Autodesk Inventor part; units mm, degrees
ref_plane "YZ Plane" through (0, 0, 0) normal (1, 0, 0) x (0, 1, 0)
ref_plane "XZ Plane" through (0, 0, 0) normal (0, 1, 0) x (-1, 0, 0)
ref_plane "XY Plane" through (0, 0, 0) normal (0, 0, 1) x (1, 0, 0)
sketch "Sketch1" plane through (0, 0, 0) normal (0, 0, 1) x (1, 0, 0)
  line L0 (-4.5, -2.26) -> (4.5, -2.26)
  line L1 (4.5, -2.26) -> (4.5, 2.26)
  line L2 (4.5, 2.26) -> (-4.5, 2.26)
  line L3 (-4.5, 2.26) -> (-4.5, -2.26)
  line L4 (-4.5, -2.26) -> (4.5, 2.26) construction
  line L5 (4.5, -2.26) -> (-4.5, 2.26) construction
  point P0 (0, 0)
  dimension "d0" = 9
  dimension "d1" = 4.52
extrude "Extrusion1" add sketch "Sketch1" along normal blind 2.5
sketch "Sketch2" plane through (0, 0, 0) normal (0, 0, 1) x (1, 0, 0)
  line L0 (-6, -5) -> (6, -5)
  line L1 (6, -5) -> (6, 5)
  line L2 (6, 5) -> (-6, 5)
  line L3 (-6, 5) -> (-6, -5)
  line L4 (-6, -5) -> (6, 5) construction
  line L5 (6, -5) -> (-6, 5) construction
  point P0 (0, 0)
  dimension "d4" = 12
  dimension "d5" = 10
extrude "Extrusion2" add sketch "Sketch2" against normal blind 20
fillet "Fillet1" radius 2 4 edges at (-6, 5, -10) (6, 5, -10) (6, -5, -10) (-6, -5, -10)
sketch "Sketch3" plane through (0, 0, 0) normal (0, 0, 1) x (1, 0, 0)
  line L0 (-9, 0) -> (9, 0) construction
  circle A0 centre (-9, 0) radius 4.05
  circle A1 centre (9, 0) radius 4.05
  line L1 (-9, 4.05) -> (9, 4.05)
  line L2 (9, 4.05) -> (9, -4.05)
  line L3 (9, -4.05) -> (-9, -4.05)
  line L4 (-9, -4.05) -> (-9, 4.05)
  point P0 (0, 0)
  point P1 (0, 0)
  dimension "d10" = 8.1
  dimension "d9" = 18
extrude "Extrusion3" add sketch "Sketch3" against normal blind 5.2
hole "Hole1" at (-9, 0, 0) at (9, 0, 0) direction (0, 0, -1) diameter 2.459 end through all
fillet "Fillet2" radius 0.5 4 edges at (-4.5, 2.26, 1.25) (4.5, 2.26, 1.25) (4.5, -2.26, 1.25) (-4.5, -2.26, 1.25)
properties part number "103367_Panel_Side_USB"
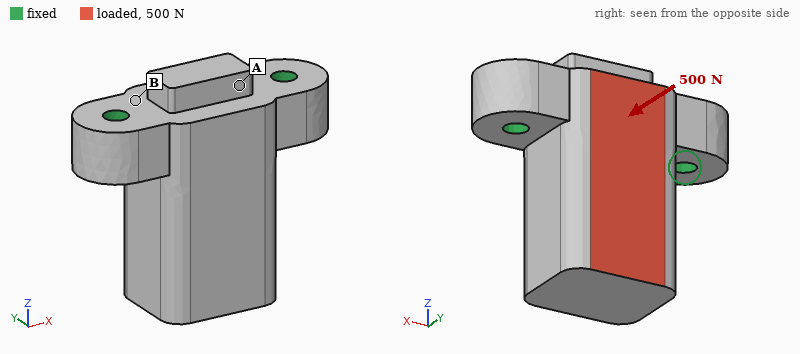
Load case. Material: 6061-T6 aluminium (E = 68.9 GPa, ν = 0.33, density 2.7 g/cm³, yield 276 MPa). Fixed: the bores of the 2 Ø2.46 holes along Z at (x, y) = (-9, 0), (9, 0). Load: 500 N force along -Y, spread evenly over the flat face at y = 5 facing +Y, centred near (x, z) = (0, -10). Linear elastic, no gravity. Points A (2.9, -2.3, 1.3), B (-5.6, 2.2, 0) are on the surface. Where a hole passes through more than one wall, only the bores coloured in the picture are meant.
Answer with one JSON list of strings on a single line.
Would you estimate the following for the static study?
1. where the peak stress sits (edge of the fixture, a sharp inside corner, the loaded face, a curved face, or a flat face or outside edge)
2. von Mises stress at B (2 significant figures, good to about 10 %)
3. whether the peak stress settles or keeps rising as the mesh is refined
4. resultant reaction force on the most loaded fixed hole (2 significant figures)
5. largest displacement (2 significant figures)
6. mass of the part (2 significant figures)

["edge of the fixture", "24 MPa", "keeps rising", "250 N", "29 µm", "7.8 g"]
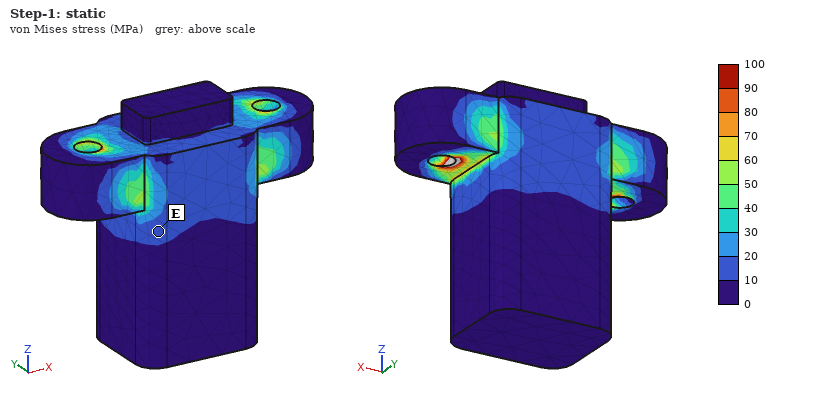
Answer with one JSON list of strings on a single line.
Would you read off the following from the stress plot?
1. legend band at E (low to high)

["10 to 20 MPa"]
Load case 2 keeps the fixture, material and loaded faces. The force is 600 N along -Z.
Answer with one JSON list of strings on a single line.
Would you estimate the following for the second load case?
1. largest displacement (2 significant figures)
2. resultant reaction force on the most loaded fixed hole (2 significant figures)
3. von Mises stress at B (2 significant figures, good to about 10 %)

["23 µm", "310 N", "31 MPa"]
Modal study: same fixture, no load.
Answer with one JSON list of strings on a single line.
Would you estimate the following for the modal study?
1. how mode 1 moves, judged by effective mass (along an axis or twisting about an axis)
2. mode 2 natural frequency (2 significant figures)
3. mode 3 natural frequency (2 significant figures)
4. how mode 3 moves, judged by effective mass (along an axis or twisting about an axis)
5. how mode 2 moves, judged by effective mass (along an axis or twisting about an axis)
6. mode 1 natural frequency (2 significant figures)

["along Y", "21 kHz", "34 kHz", "along Z", "along X", "10 kHz"]
